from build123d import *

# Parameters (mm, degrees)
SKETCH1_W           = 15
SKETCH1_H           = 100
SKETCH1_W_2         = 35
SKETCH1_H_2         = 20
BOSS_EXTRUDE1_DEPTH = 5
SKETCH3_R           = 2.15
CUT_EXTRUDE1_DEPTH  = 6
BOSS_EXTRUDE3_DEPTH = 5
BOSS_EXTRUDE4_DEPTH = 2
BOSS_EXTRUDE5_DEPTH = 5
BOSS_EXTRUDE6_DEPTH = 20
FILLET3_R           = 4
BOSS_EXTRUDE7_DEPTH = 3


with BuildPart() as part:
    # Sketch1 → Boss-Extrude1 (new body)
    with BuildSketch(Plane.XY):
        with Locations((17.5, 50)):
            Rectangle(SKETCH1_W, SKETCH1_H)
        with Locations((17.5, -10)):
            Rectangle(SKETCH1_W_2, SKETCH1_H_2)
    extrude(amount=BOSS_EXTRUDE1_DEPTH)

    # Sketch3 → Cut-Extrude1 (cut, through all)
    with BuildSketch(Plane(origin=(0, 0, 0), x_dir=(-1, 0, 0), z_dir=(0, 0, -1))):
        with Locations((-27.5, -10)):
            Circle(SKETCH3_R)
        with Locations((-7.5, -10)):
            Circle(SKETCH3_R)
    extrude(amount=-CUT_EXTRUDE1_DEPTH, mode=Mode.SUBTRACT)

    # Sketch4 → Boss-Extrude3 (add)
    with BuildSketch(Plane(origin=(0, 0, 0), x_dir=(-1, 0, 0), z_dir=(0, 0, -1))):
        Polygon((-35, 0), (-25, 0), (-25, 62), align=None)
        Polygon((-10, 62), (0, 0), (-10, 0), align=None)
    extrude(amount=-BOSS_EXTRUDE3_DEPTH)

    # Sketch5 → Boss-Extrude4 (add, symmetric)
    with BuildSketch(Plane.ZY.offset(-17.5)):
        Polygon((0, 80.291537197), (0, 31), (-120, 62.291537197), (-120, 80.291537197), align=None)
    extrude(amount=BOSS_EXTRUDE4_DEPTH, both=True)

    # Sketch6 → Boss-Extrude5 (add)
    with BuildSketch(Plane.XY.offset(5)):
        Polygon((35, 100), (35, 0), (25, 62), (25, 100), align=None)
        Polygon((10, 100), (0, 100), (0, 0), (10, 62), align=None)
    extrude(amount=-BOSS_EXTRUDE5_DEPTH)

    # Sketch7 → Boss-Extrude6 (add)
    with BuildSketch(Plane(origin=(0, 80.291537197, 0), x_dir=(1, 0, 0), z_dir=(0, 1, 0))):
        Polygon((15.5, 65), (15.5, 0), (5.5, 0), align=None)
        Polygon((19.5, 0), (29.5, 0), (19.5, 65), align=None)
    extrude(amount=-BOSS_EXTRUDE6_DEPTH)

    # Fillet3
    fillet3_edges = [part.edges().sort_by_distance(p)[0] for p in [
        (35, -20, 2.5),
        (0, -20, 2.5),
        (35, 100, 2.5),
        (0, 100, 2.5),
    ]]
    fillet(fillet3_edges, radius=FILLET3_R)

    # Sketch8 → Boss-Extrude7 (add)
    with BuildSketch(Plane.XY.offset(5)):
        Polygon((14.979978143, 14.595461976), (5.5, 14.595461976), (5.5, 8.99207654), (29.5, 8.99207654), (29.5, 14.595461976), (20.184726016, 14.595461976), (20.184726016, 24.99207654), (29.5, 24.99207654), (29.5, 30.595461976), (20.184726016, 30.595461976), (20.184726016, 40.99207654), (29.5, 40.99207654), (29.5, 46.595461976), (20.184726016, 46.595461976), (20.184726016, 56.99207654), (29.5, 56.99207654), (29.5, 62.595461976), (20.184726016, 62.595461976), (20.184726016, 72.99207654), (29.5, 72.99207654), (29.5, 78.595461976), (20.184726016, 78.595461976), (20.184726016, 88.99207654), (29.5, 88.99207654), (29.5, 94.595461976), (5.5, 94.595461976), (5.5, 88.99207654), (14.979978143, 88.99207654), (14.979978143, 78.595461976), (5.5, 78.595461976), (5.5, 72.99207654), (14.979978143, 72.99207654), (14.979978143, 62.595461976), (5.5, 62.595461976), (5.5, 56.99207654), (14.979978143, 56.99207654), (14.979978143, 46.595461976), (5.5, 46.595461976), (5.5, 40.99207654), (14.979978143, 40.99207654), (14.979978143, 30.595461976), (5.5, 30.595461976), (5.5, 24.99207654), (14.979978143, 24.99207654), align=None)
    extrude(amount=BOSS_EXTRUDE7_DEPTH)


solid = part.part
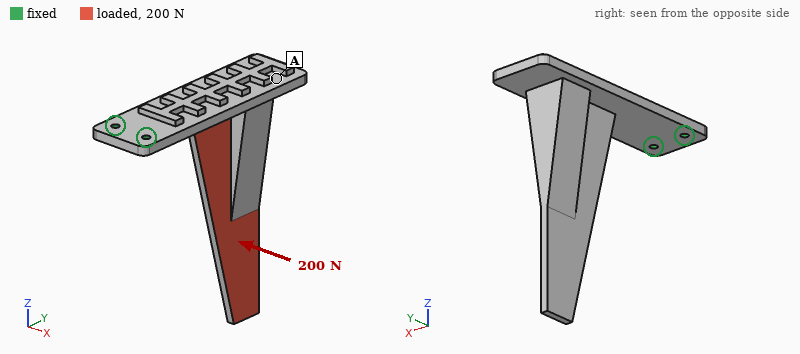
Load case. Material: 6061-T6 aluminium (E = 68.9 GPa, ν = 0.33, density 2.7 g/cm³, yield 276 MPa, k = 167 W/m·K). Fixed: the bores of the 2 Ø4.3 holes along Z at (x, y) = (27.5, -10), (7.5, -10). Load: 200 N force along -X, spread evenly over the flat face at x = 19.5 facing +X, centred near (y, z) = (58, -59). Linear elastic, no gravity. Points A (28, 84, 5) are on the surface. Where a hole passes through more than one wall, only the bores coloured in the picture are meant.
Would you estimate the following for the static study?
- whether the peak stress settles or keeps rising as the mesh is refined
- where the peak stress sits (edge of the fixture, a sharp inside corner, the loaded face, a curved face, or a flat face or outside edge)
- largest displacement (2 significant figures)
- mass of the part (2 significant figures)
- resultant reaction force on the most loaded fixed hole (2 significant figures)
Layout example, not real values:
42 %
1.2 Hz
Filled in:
keeps rising
edge of the fixture
2.0 mm
140 g
800 N
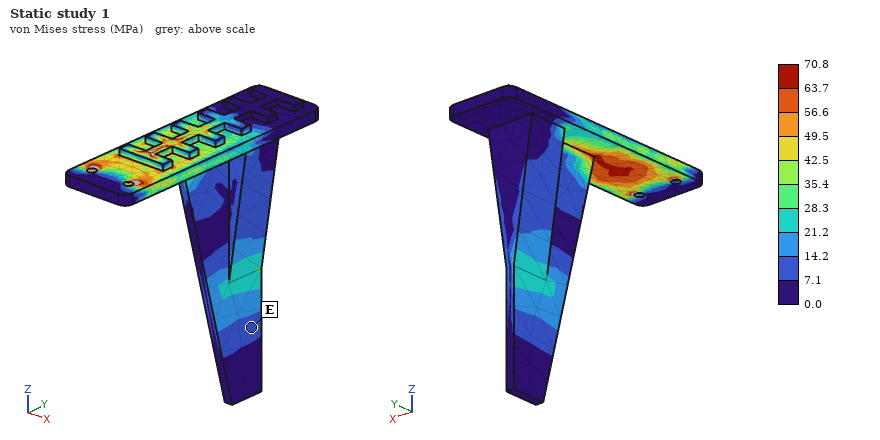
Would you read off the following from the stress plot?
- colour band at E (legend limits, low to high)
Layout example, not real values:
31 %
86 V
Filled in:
7.1 to 14.2 MPa
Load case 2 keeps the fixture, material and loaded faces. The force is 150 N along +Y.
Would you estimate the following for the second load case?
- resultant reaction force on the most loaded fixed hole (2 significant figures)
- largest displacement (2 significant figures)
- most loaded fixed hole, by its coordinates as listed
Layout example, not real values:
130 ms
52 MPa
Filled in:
91 N
1.9 mm
(27.5, -10)
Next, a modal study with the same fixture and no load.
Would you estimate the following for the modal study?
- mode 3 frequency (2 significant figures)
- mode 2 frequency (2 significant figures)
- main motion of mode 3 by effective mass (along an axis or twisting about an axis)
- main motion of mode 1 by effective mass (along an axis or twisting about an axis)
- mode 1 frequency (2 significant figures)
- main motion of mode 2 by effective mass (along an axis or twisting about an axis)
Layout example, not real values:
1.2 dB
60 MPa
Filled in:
1300 Hz
320 Hz
along X
along Z
170 Hz
along X
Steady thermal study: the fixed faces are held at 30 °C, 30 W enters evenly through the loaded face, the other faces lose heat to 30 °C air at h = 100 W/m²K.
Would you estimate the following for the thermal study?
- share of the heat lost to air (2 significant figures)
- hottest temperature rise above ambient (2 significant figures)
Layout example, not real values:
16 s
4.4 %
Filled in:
81 %
37 K
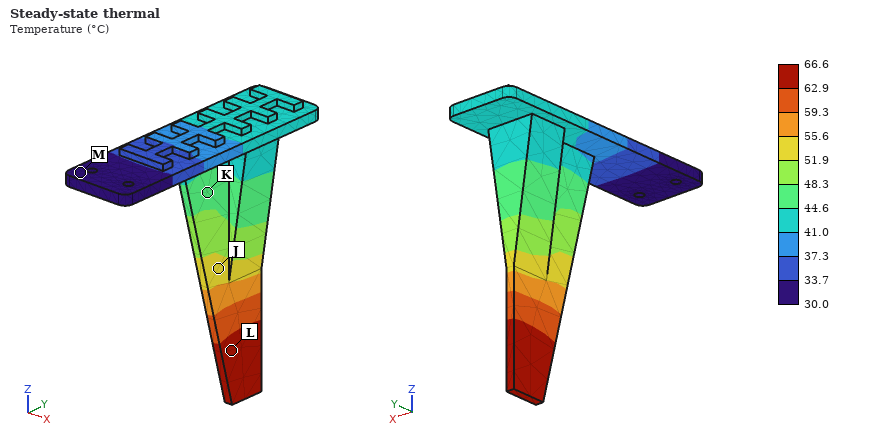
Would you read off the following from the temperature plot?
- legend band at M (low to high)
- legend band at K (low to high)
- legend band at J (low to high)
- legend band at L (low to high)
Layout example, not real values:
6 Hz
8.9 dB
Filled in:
30.0 to 33.7 °C
44.6 to 48.3 °C
51.9 to 55.6 °C
62.9 to 66.6 °C
